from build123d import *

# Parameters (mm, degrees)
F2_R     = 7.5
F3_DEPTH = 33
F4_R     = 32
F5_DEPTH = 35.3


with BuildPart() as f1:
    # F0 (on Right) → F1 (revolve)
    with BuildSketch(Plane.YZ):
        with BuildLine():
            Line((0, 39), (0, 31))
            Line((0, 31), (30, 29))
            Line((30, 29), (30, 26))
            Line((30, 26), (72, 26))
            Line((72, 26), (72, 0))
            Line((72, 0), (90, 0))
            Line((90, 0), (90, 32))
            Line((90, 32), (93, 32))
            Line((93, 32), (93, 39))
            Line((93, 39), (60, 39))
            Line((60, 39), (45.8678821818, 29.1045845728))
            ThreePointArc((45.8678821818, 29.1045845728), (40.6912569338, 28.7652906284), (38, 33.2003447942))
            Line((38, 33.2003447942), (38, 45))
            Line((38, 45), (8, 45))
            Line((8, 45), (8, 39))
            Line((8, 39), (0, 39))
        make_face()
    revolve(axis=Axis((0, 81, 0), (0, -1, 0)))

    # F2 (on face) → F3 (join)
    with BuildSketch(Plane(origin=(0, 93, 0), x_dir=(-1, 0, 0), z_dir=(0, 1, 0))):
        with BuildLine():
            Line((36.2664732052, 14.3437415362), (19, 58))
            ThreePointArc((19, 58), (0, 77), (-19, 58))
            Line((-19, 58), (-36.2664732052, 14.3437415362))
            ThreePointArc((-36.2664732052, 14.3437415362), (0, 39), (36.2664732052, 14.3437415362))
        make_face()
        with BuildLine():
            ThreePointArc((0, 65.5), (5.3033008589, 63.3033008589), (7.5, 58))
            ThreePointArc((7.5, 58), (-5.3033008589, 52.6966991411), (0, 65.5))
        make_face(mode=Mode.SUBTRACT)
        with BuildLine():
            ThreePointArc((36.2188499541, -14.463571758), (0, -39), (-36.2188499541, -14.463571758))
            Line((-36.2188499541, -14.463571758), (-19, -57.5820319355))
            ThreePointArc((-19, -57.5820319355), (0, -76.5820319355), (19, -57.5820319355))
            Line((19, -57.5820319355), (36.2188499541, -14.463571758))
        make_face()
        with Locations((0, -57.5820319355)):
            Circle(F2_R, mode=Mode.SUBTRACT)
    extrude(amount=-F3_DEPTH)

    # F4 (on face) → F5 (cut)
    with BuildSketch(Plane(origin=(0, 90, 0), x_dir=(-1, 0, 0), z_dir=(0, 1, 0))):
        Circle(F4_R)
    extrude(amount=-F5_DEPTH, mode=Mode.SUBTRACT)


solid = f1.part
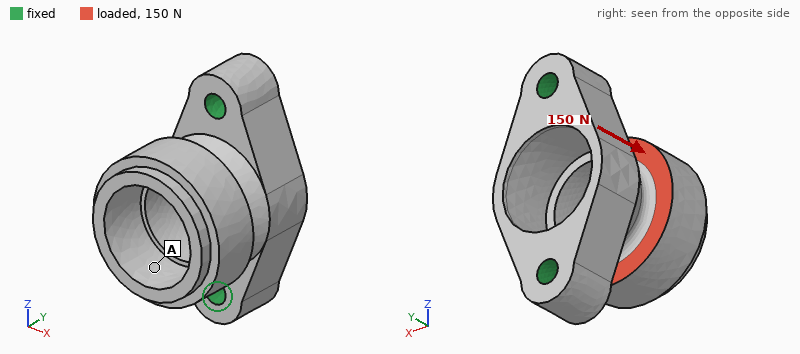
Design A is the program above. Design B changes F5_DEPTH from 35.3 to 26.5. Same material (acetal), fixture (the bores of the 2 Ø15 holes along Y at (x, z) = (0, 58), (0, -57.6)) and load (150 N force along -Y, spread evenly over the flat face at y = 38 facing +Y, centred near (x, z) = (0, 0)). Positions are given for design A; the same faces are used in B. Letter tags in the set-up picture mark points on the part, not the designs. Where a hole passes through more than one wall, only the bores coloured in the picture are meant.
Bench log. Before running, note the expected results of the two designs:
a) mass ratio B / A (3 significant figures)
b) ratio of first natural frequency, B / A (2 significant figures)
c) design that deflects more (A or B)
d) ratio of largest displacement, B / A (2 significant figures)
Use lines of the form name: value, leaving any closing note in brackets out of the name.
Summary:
mass ratio B / A: 1.03
ratio of first natural frequency, B / A: 1.0
design that deflects more: A
ratio of largest displacement, B / A: 0.77
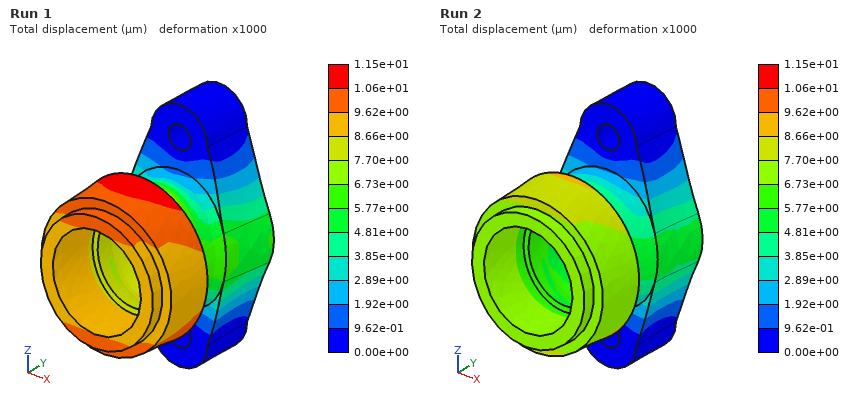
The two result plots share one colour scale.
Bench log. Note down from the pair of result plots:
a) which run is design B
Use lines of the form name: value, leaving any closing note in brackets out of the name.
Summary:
which run is design B: Run 2
